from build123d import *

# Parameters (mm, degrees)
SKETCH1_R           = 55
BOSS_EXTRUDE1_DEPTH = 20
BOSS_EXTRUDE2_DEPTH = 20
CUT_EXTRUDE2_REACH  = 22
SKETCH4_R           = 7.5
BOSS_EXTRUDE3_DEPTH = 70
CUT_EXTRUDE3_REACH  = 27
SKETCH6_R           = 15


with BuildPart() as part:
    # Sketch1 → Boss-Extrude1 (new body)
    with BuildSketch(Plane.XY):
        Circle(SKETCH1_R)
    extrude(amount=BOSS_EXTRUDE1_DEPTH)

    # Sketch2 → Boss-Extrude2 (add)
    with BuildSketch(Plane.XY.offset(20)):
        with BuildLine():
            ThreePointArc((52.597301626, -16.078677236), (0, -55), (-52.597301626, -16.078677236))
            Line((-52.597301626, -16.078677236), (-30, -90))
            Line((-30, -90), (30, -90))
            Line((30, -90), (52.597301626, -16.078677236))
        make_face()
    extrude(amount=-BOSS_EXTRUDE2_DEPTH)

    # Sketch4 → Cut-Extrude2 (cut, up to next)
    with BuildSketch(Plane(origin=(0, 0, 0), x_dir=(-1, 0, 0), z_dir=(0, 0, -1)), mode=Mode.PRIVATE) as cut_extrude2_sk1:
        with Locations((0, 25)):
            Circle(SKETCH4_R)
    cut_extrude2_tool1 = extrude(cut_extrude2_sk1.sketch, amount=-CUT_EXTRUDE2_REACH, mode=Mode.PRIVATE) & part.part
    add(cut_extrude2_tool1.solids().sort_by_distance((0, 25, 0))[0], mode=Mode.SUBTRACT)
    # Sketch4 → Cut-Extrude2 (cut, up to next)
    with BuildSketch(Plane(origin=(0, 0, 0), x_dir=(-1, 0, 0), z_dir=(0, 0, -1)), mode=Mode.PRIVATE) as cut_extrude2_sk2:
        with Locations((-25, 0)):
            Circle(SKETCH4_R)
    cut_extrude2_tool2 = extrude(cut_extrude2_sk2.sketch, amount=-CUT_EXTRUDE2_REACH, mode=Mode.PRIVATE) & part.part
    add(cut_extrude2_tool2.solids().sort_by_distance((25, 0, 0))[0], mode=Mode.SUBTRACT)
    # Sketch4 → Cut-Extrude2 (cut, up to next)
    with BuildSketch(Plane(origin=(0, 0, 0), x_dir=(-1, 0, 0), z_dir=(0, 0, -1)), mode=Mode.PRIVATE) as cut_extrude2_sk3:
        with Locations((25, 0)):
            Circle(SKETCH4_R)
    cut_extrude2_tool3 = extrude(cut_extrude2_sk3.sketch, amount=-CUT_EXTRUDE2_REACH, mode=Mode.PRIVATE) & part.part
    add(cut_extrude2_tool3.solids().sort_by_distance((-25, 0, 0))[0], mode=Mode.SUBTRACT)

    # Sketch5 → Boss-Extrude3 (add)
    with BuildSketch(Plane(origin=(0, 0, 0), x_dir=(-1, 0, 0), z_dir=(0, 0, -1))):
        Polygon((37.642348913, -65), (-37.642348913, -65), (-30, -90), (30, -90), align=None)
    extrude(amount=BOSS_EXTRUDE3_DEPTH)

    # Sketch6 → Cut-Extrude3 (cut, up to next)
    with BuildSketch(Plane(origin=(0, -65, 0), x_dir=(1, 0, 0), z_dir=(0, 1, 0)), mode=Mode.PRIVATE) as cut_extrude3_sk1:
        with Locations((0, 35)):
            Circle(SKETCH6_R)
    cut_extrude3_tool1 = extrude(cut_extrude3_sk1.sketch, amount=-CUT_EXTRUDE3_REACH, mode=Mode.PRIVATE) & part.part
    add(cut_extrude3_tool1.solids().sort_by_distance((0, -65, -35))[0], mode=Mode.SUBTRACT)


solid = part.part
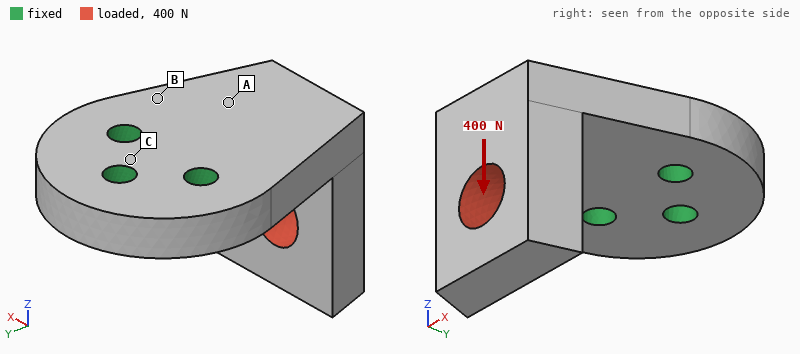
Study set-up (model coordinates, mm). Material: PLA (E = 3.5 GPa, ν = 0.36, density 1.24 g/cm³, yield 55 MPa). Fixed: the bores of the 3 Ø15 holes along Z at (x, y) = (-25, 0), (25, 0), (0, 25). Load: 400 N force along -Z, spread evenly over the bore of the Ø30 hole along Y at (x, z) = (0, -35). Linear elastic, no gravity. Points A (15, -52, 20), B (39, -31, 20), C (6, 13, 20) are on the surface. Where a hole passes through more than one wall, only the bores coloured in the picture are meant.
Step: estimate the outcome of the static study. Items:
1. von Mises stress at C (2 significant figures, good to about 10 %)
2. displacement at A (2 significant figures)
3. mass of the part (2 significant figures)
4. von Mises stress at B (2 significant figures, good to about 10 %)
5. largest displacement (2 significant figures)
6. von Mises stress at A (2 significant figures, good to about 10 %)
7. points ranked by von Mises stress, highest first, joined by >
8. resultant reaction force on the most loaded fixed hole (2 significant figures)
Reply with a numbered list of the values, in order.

1. 0.73 MPa
2. 0.14 mm
3. 420 g
4. 2.9 MPa
5. 0.53 mm
6. 1.7 MPa
7. B > A > C
8. 260 N
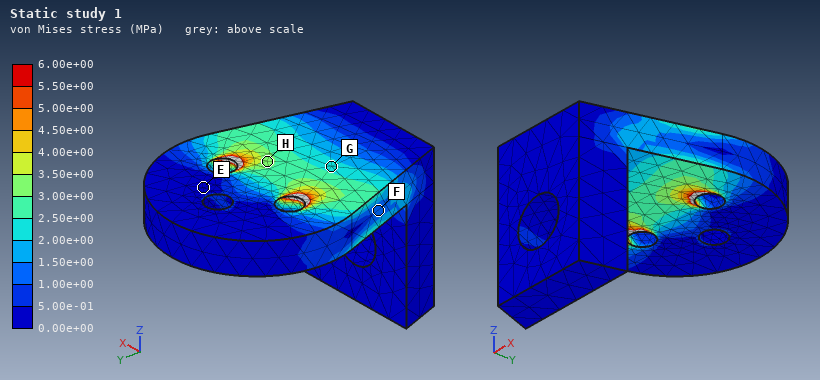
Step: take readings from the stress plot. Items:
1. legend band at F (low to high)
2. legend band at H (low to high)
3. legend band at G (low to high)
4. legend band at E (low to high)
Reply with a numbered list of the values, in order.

1. 1.00e+00 to 1.50e+00 MPa
2. 3.00e+00 to 3.50e+00 MPa
3. 2.00e+00 to 2.50e+00 MPa
4. 0.00e+00 to 5.00e-01 MPa
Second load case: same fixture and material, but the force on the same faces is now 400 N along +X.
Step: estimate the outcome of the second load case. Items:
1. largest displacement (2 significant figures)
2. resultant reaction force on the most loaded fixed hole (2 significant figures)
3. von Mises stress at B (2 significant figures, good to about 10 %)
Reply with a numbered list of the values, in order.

1. 0.30 mm
2. 590 N
3. 1.6 MPa
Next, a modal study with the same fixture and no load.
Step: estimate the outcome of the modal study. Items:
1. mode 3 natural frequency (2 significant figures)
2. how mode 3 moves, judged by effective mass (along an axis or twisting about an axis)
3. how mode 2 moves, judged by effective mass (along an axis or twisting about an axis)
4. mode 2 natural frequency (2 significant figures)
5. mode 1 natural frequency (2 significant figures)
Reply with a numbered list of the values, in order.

1. 940 Hz
2. along Z
3. along X
4. 580 Hz
5. 340 Hz
